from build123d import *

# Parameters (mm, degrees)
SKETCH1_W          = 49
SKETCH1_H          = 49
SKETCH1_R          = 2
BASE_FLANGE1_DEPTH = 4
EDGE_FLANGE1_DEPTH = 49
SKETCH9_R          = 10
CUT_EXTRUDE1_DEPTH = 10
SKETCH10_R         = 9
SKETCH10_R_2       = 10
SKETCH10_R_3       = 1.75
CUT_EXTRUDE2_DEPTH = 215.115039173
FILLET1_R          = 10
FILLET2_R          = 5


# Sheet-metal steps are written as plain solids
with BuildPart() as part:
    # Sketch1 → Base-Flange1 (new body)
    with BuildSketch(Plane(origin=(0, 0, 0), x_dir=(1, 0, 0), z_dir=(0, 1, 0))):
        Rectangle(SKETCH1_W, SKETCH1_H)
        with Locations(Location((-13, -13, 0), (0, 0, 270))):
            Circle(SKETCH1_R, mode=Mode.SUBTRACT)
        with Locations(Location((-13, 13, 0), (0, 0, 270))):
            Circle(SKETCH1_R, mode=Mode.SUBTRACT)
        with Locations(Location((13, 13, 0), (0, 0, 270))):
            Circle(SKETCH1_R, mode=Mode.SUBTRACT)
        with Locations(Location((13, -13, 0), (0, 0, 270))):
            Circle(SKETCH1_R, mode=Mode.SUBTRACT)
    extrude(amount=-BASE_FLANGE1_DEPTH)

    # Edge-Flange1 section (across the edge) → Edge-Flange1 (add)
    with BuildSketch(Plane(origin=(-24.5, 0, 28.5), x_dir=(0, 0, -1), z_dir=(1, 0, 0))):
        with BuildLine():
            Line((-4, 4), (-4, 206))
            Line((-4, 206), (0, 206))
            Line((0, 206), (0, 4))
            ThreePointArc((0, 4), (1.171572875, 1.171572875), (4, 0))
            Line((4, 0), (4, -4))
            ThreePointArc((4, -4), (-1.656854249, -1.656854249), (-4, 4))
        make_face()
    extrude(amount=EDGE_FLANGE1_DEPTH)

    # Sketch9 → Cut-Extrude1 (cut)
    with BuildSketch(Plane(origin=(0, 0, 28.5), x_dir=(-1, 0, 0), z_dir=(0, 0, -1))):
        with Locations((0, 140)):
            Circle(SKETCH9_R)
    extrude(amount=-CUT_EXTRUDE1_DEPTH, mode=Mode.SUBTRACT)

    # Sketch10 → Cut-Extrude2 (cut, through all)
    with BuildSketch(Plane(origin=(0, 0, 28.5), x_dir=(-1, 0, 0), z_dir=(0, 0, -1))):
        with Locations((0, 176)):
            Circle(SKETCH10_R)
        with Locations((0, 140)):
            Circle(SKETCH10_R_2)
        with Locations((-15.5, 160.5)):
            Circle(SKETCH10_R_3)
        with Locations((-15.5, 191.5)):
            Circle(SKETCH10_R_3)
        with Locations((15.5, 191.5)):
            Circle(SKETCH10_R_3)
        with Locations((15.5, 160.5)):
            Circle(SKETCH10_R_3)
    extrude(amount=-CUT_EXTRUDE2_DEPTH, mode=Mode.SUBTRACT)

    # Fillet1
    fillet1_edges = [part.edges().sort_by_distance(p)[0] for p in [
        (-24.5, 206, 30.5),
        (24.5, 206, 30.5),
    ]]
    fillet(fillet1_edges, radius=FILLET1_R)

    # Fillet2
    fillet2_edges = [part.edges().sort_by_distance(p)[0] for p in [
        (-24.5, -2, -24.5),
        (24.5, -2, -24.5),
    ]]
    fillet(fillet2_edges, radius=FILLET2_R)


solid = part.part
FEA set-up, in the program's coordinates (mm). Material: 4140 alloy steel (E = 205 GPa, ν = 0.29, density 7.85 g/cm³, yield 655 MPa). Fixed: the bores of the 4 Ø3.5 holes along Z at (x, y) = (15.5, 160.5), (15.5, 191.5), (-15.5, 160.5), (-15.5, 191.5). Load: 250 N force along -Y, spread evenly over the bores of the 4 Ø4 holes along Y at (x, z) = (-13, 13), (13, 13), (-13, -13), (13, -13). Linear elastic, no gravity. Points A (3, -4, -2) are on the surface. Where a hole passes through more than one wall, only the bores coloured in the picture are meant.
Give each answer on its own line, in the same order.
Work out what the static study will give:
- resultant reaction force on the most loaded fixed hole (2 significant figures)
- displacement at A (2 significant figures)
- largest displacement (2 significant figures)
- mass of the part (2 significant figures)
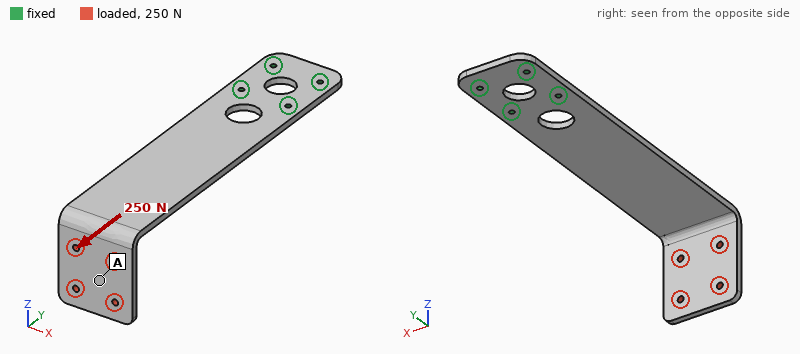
110 N
2.4 mm
2.7 mm
380 g
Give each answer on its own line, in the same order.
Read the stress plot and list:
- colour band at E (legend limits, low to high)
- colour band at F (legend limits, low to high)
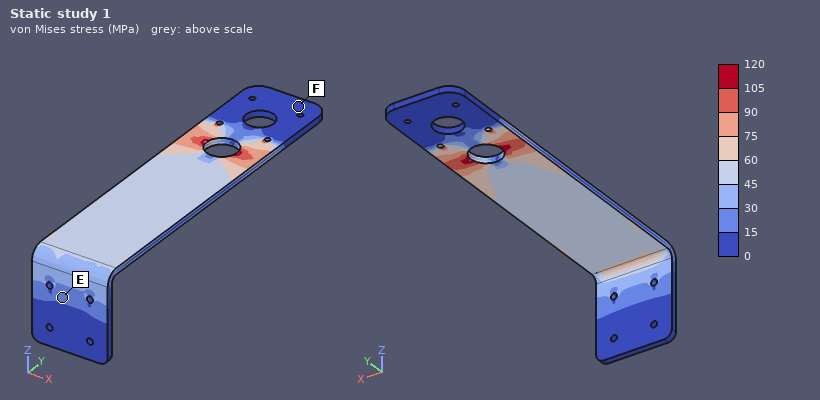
15 to 30 MPa
0 to 15 MPa
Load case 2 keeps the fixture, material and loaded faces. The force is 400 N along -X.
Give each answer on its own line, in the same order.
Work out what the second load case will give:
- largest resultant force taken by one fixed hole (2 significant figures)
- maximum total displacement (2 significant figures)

1.7 kN
1.5 mm
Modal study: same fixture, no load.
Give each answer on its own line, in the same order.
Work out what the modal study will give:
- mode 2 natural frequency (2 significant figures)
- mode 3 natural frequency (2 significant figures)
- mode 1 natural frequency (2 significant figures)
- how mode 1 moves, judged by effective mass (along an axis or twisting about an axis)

330 Hz
430 Hz
73 Hz
along Z
